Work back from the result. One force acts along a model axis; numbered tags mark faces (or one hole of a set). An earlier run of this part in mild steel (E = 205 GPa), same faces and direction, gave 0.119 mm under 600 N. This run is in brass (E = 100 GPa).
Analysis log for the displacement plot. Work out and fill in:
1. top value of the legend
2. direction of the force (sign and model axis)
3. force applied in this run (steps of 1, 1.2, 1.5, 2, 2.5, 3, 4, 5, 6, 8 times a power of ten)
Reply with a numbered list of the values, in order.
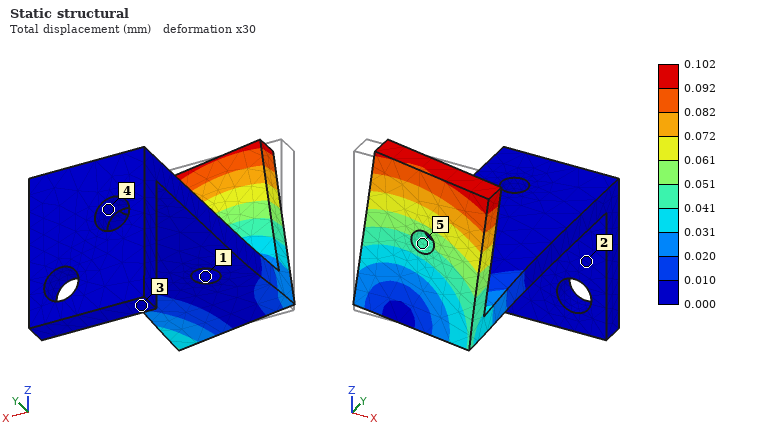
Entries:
1. 0.102 mm
2. +X
3. 250 N
